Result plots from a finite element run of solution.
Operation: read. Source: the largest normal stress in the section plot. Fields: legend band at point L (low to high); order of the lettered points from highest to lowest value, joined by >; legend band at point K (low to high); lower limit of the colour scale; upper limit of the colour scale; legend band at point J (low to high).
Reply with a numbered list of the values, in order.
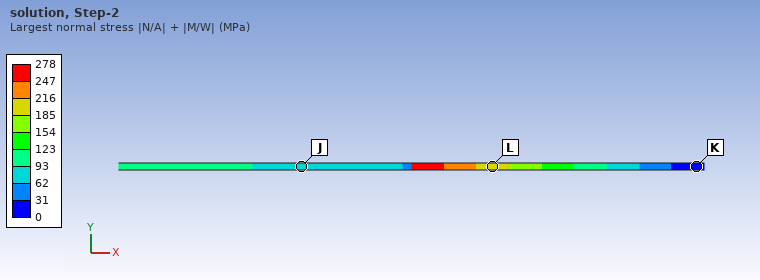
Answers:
1. 185 to 216 MPa
2. L > J > K
3. 0 to 31 MPa
4. 0 MPa
5. 278 MPa
6. 62 to 93 MPa
